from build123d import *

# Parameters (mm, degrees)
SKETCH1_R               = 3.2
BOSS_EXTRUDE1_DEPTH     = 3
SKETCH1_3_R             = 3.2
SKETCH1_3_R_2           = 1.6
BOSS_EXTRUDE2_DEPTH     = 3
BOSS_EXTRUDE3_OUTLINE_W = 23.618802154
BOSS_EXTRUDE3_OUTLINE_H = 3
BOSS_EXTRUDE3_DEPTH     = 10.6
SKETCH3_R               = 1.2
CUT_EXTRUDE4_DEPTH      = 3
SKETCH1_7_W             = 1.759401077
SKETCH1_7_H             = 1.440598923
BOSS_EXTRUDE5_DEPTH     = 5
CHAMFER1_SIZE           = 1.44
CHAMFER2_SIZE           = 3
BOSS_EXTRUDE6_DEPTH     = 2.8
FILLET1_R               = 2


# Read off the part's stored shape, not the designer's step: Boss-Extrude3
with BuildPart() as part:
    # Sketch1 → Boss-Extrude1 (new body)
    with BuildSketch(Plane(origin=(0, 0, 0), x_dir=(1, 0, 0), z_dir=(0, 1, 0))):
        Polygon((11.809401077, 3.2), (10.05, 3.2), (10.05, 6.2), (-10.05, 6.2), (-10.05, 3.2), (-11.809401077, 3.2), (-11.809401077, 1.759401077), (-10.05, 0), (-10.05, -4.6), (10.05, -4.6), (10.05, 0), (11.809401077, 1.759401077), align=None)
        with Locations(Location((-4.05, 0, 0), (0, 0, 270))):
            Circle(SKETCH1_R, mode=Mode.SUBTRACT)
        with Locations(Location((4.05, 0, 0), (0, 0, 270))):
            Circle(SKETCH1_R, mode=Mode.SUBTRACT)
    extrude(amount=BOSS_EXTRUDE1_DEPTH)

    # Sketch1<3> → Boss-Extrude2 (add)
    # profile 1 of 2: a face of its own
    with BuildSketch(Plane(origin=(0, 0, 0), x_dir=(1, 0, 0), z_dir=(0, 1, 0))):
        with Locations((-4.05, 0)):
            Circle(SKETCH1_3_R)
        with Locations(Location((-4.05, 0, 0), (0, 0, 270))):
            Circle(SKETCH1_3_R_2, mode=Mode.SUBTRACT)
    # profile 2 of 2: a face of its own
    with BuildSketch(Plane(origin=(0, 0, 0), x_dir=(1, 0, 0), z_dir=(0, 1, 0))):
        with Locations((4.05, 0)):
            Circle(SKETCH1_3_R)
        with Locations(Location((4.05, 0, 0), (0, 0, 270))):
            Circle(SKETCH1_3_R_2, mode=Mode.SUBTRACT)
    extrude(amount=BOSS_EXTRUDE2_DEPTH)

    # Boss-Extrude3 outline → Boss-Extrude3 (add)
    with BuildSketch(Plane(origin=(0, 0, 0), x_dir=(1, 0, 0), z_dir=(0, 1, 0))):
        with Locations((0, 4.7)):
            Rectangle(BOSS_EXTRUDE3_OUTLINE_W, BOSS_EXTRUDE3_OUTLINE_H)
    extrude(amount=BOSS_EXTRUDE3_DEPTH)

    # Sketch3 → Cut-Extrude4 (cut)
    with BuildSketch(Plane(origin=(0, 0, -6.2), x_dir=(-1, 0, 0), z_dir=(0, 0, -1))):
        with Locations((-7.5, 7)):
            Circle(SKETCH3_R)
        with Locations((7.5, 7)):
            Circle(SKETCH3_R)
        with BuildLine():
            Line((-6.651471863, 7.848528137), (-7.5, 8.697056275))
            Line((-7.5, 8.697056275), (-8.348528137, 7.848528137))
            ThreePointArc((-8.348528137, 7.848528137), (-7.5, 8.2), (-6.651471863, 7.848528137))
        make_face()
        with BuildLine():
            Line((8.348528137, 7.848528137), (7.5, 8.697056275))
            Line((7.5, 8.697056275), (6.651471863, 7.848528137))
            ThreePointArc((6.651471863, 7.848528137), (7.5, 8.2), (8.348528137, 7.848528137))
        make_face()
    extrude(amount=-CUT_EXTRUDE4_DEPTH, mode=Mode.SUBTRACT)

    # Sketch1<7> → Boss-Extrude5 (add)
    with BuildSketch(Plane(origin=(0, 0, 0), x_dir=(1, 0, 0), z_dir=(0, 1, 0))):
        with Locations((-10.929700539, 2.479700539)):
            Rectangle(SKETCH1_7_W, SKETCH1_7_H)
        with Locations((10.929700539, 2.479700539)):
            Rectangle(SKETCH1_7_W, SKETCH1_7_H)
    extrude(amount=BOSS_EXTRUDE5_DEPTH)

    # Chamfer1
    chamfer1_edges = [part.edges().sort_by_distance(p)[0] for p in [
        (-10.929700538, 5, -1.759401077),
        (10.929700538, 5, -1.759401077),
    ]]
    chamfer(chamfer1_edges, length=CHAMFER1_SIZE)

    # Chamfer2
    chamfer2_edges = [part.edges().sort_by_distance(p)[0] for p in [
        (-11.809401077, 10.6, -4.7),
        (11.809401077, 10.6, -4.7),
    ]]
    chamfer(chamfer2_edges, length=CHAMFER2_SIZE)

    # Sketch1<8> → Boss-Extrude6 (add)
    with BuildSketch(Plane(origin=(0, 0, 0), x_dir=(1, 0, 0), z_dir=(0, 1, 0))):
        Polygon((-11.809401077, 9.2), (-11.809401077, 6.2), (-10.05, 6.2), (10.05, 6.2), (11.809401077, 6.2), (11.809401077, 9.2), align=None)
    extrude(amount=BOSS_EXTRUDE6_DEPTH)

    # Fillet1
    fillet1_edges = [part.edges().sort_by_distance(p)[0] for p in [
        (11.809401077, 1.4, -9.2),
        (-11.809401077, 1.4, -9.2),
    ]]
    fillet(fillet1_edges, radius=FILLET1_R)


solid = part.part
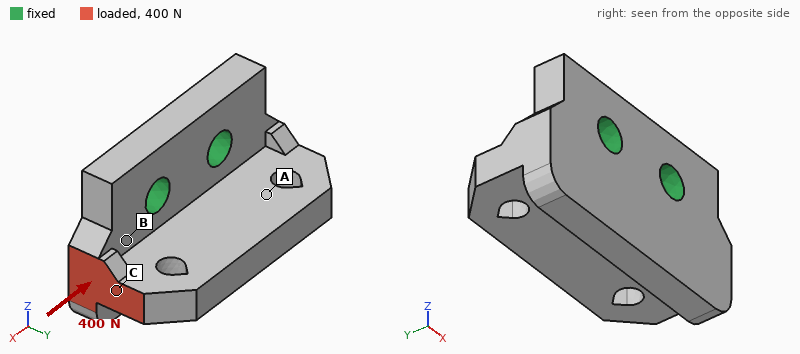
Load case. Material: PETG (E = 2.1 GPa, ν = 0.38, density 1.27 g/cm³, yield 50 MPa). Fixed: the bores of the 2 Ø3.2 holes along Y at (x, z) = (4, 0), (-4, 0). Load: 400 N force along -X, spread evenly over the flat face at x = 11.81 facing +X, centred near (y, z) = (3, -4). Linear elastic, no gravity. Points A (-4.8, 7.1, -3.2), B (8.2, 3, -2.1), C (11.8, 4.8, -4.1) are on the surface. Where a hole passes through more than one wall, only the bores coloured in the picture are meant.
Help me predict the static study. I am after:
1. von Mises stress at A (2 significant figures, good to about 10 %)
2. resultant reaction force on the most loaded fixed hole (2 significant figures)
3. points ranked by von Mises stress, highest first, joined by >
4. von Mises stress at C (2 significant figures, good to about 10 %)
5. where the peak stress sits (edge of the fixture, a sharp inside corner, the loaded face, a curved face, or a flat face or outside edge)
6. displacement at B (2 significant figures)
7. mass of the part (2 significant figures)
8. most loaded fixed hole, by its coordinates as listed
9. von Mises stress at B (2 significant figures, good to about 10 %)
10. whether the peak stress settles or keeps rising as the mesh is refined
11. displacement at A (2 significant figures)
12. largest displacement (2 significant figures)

4.3 MPa
290 N
B > C > A
11 MPa
edge of the fixture
0.056 mm
1.7 g
(4, 0)
19 MPa
keeps rising
0.077 mm
0.16 mm
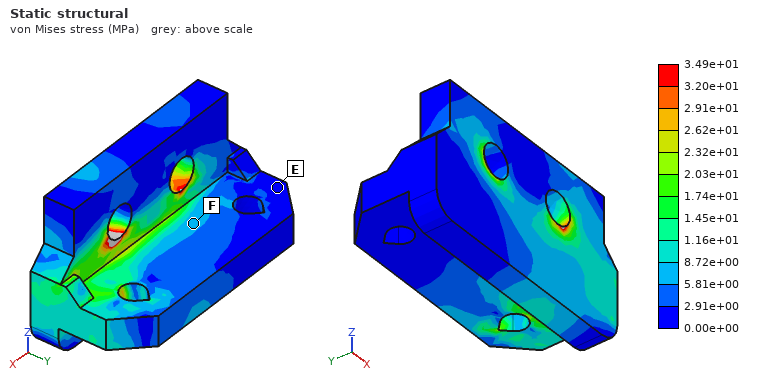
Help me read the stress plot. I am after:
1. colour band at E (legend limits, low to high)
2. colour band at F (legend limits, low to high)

0.00e+00 to 2.91e+00 MPa
5.81e+00 to 8.72e+00 MPa
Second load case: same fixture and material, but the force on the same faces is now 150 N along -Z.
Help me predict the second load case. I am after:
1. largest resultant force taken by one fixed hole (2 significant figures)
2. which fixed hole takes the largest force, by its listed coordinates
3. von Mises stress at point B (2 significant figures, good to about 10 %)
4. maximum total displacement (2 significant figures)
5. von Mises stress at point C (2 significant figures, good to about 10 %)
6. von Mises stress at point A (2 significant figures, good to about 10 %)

240 N
(4, 0)
19 MPa
0.28 mm
23 MPa
2.9 MPa
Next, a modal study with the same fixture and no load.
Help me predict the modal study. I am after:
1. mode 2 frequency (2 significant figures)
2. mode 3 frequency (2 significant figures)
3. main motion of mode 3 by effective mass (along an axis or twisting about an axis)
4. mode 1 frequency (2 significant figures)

5600 Hz
8800 Hz
along X
4300 Hz
